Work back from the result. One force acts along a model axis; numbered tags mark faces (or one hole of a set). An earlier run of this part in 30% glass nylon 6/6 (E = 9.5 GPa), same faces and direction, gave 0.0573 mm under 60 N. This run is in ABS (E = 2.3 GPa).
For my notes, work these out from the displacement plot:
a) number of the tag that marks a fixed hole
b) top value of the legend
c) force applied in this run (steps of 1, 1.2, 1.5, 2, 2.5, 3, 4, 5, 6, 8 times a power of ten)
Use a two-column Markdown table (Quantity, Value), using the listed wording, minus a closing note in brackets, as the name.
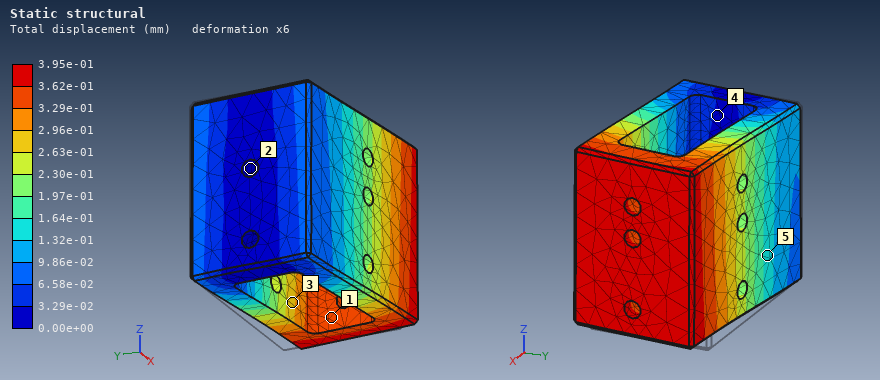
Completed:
| Quantity | Value |
|---|---|
| number of the tag that marks a fixed hole | 2 |
| top value of the legend | 3.95e-01 mm |
| force applied in this run | 100 N |
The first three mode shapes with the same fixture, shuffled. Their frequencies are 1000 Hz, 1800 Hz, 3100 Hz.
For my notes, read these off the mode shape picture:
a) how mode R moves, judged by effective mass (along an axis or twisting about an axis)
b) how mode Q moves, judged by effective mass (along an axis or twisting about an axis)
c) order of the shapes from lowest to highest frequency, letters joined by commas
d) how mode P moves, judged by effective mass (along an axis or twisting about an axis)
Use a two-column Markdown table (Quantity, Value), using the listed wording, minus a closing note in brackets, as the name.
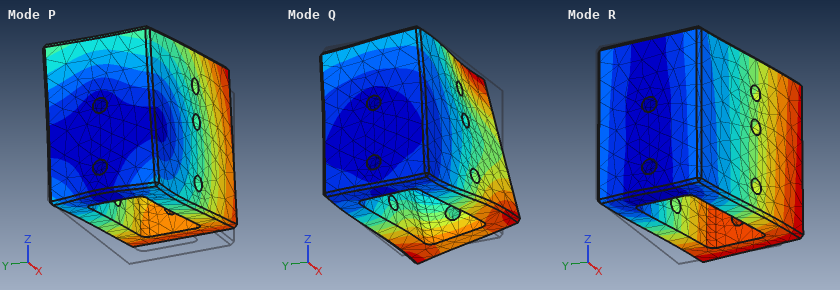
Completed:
| Quantity | Value |
|---|---|
| how mode R moves, judged by effective mass | along Y |
| how mode Q moves, judged by effective mass | twisting about X |
| order of the shapes from lowest to highest frequency, letters joined by commas | R, P, Q |
| how mode P moves, judged by effective mass | along Z |
